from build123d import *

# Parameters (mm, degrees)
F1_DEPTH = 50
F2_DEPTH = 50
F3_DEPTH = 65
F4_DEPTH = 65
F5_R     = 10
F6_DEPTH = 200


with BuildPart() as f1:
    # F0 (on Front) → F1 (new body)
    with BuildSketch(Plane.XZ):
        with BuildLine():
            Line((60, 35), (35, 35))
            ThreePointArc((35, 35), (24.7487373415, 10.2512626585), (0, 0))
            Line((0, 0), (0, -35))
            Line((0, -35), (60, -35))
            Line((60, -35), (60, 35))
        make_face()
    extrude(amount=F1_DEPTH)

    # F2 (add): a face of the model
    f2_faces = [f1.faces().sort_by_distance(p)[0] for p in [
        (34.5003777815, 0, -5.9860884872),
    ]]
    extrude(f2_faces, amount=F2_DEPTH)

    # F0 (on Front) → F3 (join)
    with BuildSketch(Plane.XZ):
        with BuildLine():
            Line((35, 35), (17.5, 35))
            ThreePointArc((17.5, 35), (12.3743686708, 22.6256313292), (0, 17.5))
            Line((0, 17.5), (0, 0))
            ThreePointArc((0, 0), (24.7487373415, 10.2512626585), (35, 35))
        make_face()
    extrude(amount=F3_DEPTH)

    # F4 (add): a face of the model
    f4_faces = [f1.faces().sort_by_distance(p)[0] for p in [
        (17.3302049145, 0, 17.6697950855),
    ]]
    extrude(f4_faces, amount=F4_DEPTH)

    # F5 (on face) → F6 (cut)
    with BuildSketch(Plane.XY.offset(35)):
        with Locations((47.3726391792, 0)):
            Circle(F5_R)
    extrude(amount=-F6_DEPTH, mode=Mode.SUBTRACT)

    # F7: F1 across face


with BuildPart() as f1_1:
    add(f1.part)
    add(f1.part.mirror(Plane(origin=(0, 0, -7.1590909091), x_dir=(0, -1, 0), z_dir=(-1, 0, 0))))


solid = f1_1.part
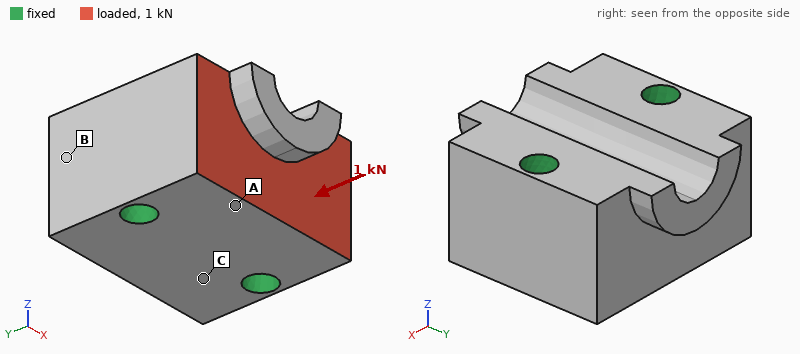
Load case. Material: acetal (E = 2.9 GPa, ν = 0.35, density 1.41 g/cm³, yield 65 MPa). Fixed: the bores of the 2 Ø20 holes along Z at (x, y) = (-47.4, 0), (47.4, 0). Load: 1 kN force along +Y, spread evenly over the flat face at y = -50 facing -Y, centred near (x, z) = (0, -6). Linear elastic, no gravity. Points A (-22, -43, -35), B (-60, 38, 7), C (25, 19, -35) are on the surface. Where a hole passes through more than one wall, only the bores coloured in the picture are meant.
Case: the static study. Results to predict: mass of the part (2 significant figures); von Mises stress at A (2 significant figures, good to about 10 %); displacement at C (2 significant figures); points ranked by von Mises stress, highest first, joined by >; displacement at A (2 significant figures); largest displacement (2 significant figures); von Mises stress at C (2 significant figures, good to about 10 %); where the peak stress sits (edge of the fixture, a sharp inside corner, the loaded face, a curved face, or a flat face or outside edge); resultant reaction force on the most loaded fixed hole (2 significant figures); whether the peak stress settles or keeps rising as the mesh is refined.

1.1 kg
0.15 MPa
1.2 µm
A > C > B
3.5 µm
4.4 µm
0.085 MPa
edge of the fixture
500 N
keeps rising
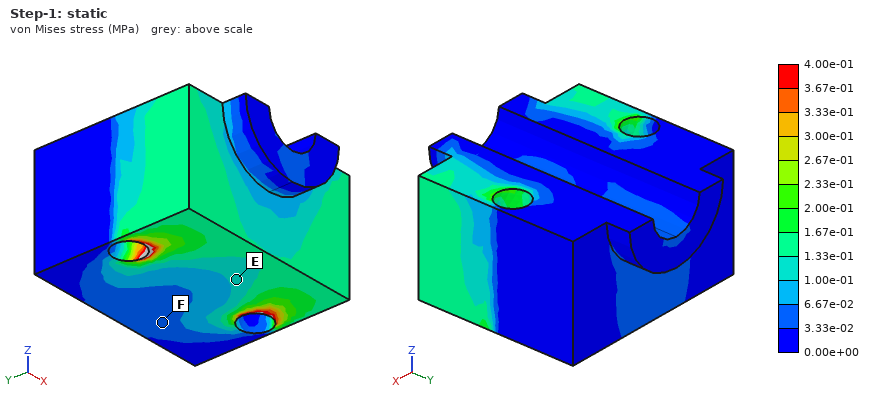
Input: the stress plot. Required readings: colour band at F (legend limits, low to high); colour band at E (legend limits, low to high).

3.33e-02 to 6.67e-02 MPa
1.00e-01 to 1.33e-01 MPa
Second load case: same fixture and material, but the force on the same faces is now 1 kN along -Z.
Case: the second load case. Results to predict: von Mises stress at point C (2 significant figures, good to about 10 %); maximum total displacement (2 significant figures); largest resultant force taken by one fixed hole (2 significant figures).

0.16 MPa
16 µm
500 N
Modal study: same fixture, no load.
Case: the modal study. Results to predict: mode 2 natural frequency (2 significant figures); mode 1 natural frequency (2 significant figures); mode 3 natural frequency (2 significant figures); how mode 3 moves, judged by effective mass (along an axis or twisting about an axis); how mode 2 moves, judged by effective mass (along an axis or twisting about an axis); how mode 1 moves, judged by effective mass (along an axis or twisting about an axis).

2900 Hz
2700 Hz
3500 Hz
along X
along Z
twisting about X
